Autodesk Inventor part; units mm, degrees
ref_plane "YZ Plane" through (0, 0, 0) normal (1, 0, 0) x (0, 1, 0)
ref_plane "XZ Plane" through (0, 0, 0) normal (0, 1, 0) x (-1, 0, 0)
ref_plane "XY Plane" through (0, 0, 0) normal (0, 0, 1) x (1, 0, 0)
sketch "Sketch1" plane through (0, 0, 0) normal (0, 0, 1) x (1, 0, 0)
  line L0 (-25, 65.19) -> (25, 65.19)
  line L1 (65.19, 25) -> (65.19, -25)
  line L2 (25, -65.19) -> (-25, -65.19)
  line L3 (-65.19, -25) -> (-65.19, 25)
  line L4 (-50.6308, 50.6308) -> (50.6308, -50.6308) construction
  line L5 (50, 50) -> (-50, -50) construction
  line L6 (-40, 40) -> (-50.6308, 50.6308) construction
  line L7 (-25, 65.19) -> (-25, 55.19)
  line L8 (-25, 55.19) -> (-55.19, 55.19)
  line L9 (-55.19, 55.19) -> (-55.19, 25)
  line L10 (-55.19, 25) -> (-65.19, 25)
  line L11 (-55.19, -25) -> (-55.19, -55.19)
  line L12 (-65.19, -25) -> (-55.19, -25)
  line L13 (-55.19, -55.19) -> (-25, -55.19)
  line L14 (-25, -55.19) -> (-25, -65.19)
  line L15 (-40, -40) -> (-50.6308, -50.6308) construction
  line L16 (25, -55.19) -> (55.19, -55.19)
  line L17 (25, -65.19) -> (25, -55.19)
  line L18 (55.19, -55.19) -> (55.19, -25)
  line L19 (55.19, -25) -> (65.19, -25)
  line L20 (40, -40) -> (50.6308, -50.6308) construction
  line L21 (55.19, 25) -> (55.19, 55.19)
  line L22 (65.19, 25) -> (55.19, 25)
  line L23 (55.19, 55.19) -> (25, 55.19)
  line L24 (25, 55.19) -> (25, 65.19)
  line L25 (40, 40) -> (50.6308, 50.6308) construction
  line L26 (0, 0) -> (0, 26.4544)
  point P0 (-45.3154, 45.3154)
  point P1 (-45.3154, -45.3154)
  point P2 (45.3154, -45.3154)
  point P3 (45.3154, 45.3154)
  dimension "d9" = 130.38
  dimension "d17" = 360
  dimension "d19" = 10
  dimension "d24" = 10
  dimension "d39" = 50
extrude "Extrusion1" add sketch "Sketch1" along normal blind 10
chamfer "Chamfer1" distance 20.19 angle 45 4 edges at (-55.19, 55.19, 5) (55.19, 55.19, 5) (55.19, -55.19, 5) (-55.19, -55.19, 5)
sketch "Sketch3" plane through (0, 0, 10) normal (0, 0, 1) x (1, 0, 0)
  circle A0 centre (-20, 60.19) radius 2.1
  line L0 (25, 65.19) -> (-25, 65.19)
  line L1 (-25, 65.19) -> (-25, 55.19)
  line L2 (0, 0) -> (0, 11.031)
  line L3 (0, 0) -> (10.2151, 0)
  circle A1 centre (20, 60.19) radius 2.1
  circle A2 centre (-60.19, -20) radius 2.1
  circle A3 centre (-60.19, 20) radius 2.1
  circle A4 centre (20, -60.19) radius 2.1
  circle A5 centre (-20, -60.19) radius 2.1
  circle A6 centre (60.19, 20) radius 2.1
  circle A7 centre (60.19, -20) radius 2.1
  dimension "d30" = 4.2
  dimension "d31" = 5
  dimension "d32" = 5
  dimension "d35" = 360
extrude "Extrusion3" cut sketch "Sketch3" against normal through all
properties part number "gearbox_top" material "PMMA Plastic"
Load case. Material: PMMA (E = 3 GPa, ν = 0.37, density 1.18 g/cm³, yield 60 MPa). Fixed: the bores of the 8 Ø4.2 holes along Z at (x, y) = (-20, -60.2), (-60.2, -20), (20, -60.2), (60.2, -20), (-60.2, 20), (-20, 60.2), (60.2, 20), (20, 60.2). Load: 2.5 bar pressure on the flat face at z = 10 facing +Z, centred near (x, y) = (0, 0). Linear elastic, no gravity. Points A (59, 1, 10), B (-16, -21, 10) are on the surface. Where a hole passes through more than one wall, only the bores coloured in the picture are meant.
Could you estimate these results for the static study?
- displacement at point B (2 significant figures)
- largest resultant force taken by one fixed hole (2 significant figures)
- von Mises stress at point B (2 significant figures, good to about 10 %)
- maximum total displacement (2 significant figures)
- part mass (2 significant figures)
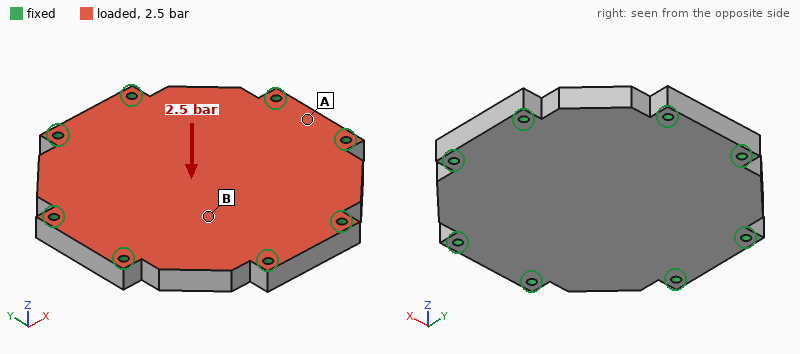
0.31 mm
410 N
5.2 MPa
0.41 mm
160 g
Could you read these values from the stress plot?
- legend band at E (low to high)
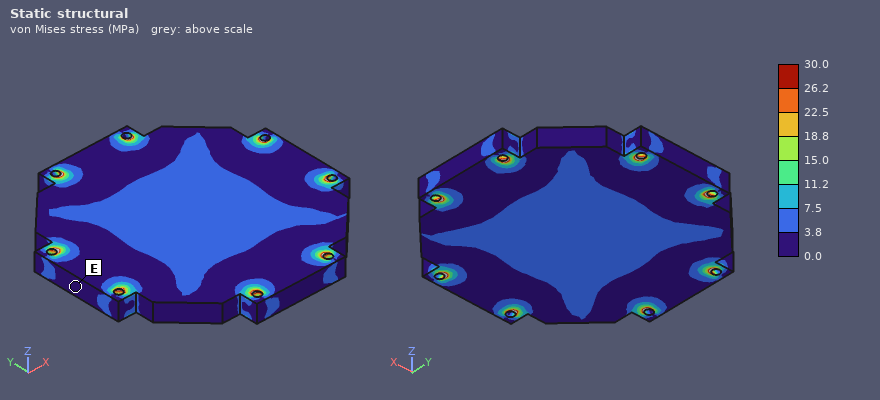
0.0 to 3.8 MPa
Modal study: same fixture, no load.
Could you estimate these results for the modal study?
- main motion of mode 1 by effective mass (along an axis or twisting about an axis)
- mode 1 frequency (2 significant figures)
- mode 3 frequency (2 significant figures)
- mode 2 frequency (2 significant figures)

along Z
1400 Hz
2900 Hz
2900 Hz
